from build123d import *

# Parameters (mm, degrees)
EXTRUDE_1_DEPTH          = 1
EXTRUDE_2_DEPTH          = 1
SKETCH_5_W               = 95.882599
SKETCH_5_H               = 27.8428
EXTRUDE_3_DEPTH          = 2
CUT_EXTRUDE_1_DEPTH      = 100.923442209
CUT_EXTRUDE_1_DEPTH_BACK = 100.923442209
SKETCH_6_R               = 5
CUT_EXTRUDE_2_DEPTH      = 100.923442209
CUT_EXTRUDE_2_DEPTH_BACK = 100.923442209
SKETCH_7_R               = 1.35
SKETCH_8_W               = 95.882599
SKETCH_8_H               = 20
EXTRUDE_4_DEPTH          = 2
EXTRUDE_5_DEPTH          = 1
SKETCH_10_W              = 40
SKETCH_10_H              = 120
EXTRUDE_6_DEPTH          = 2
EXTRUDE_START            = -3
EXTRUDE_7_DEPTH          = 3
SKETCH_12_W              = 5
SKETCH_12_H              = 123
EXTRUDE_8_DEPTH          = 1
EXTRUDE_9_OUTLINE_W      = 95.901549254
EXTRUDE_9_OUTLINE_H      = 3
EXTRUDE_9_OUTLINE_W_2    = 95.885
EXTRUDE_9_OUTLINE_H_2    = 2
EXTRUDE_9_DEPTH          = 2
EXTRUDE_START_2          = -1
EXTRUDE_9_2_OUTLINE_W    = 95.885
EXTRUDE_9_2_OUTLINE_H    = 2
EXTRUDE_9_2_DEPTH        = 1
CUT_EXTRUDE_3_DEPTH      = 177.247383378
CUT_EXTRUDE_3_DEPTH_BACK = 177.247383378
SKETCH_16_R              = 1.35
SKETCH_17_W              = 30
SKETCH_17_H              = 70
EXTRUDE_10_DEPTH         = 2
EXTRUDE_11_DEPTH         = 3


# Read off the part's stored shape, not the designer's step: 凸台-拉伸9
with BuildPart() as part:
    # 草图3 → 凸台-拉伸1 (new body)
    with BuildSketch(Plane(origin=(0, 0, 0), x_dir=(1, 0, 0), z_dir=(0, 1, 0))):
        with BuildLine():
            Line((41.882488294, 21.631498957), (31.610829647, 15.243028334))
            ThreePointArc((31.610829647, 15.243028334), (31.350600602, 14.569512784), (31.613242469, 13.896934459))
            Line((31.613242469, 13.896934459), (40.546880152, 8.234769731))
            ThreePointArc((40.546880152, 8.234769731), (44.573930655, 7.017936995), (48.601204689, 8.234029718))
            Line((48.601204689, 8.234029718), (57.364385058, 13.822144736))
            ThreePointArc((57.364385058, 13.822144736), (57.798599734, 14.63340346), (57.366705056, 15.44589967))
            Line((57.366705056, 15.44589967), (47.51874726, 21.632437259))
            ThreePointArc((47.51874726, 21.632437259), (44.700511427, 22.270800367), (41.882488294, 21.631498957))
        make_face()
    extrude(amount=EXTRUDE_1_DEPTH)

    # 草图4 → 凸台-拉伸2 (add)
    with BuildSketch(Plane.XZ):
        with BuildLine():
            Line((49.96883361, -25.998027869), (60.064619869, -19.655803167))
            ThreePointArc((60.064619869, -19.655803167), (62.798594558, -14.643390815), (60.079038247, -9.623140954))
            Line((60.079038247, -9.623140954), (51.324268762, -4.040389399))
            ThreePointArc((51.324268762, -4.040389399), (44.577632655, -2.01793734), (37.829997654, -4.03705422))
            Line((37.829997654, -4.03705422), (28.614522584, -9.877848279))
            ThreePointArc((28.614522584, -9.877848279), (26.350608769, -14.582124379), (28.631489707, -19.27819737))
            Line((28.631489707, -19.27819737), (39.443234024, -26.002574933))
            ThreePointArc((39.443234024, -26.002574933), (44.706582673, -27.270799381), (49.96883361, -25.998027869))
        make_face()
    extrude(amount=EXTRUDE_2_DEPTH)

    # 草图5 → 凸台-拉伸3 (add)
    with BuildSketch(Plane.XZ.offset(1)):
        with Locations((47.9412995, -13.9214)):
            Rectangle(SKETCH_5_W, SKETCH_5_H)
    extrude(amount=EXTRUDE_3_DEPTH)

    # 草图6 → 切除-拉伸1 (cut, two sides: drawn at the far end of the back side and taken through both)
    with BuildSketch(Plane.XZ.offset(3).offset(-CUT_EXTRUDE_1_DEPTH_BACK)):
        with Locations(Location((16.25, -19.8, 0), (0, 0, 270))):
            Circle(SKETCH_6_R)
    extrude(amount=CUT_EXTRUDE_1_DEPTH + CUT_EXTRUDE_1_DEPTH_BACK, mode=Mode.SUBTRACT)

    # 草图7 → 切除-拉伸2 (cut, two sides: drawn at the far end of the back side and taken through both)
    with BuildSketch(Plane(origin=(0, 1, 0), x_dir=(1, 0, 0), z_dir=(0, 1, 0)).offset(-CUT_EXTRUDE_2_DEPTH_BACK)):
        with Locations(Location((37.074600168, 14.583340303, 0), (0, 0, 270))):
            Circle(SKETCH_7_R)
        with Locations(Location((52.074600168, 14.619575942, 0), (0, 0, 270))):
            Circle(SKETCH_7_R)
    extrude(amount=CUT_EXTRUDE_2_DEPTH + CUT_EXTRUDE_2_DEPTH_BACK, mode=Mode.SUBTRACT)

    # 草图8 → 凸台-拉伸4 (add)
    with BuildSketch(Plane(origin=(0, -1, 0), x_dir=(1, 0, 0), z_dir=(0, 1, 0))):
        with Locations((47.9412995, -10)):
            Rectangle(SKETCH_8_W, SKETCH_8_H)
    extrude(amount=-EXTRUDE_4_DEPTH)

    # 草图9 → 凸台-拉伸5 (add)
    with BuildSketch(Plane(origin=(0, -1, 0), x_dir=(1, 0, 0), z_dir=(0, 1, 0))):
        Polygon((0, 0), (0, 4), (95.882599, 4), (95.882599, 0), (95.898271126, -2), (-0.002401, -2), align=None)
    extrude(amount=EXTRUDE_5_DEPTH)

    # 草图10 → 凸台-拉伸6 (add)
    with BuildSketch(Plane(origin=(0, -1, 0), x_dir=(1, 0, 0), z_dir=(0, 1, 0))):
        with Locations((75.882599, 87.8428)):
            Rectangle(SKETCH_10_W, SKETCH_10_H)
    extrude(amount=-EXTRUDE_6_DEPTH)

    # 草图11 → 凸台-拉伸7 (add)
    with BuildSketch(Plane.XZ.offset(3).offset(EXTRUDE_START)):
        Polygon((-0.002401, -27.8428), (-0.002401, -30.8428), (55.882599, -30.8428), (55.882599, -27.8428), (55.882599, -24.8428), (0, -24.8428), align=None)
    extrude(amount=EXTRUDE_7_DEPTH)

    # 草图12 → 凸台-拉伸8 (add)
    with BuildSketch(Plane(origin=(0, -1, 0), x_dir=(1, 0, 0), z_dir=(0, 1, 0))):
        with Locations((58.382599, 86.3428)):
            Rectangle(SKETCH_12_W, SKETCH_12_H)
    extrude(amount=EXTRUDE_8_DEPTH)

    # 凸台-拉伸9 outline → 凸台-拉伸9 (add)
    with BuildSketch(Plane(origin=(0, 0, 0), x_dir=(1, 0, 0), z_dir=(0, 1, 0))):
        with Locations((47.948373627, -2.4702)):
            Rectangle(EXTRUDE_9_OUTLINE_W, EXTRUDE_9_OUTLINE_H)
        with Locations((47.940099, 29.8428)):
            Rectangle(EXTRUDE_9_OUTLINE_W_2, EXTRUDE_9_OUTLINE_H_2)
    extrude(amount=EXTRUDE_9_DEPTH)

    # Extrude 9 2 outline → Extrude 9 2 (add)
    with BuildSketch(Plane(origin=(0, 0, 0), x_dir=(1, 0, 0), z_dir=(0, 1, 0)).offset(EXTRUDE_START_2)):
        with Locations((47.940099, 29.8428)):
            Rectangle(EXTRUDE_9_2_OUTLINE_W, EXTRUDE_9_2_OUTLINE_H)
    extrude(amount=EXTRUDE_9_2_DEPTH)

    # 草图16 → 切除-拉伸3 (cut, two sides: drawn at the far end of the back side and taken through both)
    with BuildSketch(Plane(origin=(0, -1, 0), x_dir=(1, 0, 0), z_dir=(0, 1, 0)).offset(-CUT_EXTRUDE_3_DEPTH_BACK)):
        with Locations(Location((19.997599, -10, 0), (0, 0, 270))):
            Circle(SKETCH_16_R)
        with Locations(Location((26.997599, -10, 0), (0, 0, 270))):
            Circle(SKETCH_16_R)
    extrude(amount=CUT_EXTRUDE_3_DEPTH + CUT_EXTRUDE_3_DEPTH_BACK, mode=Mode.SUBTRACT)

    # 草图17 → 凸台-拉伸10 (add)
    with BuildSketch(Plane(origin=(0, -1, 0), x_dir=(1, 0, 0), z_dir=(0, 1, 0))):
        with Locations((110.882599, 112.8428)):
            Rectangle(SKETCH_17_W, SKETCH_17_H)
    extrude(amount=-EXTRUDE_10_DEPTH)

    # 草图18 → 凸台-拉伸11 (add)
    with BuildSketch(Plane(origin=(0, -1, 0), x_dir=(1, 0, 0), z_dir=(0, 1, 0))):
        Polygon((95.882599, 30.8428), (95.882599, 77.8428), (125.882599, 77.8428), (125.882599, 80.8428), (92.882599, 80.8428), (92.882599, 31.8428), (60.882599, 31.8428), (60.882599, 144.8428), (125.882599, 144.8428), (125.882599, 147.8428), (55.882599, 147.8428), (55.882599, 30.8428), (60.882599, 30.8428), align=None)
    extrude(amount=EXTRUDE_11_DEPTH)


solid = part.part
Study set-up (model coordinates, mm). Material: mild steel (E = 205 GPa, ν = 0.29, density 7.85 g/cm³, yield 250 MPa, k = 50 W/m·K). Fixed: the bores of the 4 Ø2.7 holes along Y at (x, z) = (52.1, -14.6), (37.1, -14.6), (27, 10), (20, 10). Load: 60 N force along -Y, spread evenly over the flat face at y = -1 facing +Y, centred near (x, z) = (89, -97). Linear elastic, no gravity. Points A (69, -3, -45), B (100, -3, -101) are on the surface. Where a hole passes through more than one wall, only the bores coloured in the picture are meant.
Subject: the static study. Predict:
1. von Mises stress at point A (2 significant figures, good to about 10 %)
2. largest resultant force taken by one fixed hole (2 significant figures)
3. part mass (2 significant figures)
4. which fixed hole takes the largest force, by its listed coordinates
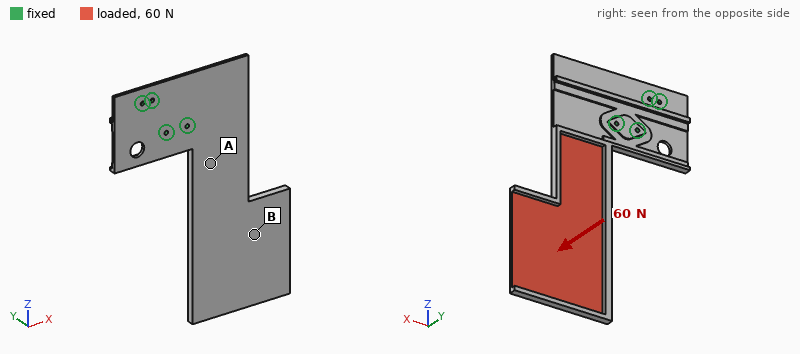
42 MPa
170 N
230 g
(52.1, -14.6)
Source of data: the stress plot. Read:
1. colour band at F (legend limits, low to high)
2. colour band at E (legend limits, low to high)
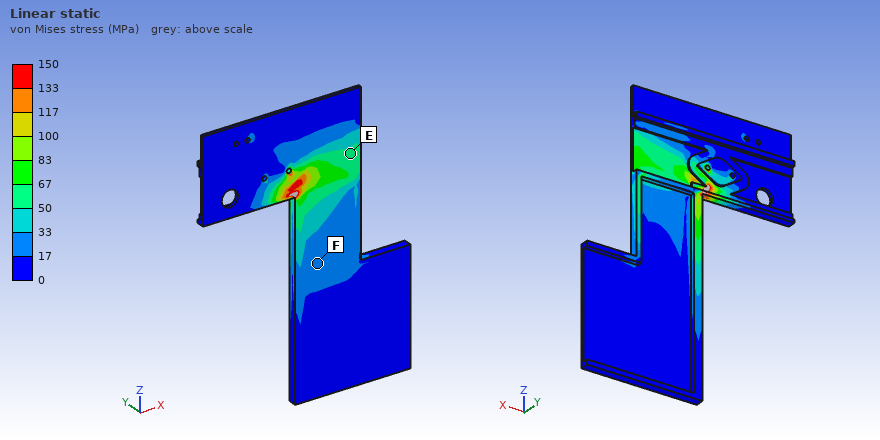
17 to 33 MPa
50 to 67 MPa
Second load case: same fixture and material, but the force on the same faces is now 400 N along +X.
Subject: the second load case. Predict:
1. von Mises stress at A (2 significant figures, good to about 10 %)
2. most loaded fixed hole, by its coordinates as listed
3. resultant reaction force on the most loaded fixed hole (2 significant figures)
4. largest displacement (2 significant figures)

16 MPa
(52.1, -14.6)
930 N
0.19 mm
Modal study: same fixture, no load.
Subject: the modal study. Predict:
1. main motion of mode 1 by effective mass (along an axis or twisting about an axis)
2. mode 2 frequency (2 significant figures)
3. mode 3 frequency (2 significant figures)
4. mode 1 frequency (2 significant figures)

along Y
370 Hz
700 Hz
100 Hz
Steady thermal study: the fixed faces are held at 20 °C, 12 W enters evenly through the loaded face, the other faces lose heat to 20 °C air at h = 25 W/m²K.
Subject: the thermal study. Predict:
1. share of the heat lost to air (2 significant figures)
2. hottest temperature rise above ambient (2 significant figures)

83 %
45 K
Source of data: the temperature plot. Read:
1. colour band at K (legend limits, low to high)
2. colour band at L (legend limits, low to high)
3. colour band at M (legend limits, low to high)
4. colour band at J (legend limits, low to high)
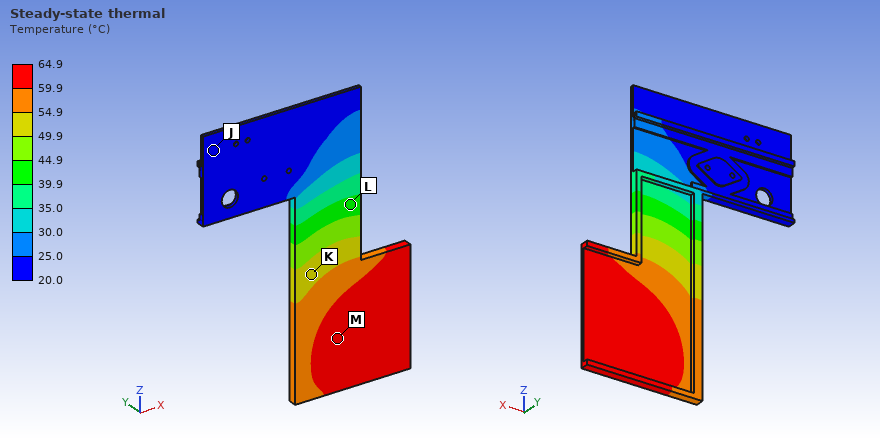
49.9 to 54.9 °C
39.9 to 44.9 °C
59.9 to 64.9 °C
20.0 to 25.0 °C
